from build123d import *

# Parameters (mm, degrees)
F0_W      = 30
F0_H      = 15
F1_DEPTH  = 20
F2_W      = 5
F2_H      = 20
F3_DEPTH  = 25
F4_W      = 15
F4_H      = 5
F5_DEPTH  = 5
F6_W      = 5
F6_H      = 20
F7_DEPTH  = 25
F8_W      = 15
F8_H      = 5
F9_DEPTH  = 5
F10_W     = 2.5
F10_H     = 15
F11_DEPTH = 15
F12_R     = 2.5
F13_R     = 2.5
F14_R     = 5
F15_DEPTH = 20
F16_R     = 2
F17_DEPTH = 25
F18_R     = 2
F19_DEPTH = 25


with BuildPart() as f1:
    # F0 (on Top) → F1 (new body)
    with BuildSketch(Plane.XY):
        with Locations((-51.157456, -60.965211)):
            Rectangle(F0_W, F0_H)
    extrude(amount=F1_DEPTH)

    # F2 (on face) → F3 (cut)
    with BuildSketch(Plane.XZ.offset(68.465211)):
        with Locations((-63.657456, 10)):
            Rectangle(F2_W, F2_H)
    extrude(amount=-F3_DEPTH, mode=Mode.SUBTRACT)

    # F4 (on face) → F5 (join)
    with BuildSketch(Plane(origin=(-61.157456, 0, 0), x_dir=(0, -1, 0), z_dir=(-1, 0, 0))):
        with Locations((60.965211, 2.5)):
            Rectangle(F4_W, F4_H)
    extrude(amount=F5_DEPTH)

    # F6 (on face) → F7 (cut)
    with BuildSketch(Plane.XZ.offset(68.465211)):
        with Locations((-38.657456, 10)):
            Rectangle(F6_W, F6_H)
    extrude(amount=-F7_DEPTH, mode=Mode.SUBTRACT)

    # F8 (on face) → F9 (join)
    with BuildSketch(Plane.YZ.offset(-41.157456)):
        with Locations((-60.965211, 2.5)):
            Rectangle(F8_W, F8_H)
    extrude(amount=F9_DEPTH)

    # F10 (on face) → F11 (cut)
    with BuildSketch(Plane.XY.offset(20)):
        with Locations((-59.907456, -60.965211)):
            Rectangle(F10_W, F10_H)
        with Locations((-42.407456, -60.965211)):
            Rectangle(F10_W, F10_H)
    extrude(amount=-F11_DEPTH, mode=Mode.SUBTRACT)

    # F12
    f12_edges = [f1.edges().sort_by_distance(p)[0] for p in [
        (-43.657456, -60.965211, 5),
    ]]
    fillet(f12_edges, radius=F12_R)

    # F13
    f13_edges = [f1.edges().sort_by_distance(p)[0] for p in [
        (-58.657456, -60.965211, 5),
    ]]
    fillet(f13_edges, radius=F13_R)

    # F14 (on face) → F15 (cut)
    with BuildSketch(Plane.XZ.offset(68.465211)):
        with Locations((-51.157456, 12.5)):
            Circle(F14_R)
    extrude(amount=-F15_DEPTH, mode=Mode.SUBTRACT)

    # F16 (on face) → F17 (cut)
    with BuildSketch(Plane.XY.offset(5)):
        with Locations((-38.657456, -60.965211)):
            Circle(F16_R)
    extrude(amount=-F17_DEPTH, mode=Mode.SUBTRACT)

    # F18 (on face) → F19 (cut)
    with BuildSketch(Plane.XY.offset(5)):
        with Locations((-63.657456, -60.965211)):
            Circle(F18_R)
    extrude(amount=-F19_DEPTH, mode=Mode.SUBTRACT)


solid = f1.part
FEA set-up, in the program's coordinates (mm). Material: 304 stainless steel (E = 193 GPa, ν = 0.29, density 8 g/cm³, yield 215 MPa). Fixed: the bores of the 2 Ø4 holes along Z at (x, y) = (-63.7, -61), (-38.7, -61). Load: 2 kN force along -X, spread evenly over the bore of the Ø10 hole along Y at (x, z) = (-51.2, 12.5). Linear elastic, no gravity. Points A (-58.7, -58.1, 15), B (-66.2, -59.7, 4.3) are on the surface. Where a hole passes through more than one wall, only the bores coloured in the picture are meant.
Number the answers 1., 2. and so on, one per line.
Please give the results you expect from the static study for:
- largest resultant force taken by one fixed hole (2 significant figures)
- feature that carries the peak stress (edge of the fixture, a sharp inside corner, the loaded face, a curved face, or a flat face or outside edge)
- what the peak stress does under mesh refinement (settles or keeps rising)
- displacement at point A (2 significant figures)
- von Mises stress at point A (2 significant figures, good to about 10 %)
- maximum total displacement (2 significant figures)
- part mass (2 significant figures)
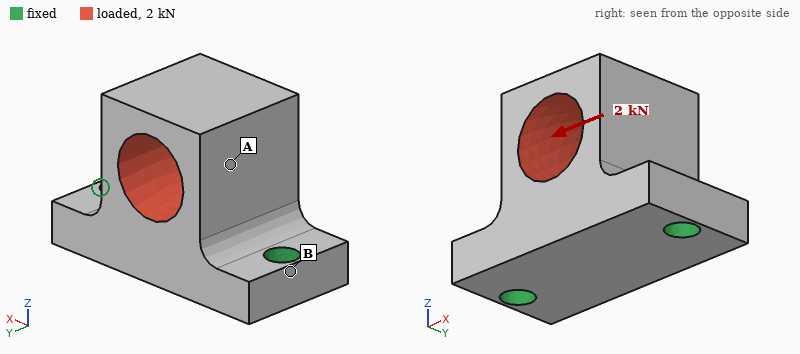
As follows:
1. 1.4 kN
2. edge of the fixture
3. keeps rising
4. 9.2 µm
5. 32 MPa
6. 12 µm
7. 35 g
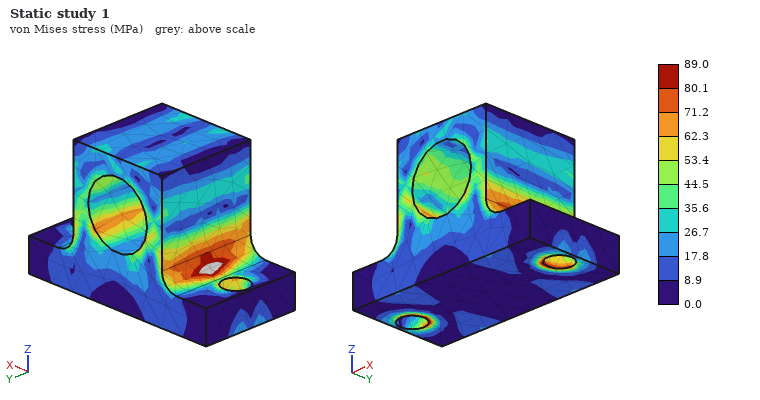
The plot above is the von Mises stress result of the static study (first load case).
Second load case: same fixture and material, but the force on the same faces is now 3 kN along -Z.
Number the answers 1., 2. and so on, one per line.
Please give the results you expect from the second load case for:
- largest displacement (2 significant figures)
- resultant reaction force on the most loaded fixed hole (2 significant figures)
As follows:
1. 5.4 µm
2. 1.6 kN
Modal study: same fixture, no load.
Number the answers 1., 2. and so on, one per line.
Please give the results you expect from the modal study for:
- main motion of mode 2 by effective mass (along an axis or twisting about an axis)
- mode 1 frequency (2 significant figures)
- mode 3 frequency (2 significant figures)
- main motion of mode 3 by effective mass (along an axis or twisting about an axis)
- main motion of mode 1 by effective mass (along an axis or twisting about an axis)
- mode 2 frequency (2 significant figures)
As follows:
1. along X
2. 11 kHz
3. 27 kHz
4. along Z
5. along Y
6. 17 kHz
